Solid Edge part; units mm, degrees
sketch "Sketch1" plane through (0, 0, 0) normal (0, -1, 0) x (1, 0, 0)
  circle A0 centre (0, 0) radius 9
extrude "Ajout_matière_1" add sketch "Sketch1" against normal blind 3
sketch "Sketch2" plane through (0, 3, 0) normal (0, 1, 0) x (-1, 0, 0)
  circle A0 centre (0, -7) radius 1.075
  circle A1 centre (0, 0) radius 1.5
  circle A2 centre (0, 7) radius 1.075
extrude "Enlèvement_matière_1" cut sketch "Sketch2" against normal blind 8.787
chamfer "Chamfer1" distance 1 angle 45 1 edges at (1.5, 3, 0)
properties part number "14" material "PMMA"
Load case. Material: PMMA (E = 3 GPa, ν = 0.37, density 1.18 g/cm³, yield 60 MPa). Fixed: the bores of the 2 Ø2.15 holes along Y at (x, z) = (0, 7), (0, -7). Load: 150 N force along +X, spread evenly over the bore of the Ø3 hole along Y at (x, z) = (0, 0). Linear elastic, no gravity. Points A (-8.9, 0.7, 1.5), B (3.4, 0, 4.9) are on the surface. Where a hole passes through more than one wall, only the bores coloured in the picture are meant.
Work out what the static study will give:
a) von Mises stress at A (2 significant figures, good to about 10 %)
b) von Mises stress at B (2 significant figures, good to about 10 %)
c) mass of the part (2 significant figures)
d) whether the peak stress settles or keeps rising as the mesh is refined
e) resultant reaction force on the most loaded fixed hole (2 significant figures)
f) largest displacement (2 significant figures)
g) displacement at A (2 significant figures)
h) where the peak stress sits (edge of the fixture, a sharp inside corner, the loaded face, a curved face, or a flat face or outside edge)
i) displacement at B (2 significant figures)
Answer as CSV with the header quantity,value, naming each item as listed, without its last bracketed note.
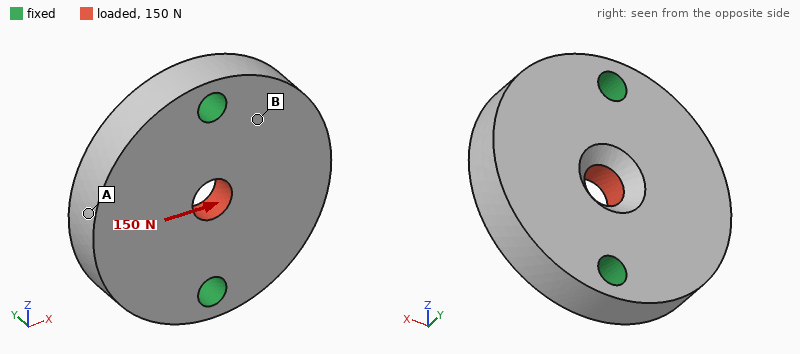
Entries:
quantity,value
von Mises stress at A,2.1 MPa
von Mises stress at B,4.1 MPa
mass of the part,0.84 g
whether the peak stress settles or keeps rising as the mesh is refined,keeps rising
resultant reaction force on the most loaded fixed hole,75 N
largest displacement,20 µm
displacement at A,17 µm
where the peak stress sits,edge of the fixture
displacement at B,8.4 µm
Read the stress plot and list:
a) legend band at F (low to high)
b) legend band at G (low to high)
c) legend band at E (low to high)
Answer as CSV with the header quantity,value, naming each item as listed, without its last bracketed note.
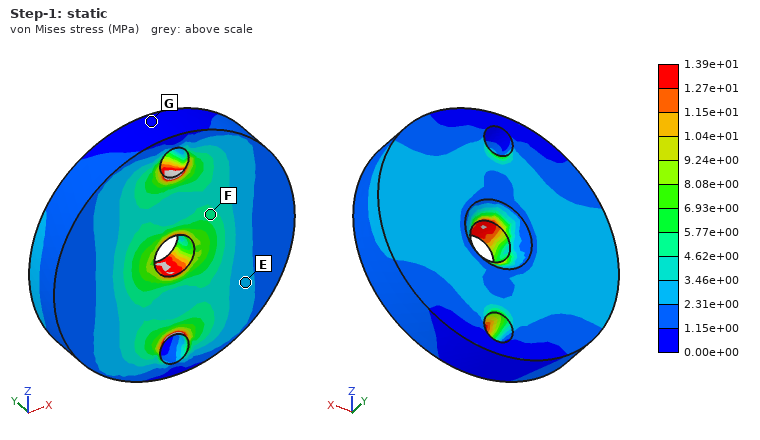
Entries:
quantity,value
legend band at F,4.62e+00 to 5.77e+00 MPa
legend band at G,0.00e+00 to 1.15e+00 MPa
legend band at E,2.31e+00 to 3.46e+00 MPa
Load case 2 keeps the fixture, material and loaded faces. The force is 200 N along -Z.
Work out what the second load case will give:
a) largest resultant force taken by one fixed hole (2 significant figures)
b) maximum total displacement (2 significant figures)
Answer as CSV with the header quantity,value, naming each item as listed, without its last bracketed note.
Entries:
quantity,value
largest resultant force taken by one fixed hole,100 N
maximum total displacement,16 µm
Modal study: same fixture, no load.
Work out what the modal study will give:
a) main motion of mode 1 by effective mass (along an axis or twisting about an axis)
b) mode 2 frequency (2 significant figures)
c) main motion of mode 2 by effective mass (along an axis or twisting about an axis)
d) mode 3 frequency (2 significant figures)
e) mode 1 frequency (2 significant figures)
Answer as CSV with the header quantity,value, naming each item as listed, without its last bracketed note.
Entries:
quantity,value
main motion of mode 1 by effective mass,twisting about Z
mode 2 frequency,10 kHz
main motion of mode 2 by effective mass,along Y
mode 3 frequency,21 kHz
mode 1 frequency,8500 Hz
